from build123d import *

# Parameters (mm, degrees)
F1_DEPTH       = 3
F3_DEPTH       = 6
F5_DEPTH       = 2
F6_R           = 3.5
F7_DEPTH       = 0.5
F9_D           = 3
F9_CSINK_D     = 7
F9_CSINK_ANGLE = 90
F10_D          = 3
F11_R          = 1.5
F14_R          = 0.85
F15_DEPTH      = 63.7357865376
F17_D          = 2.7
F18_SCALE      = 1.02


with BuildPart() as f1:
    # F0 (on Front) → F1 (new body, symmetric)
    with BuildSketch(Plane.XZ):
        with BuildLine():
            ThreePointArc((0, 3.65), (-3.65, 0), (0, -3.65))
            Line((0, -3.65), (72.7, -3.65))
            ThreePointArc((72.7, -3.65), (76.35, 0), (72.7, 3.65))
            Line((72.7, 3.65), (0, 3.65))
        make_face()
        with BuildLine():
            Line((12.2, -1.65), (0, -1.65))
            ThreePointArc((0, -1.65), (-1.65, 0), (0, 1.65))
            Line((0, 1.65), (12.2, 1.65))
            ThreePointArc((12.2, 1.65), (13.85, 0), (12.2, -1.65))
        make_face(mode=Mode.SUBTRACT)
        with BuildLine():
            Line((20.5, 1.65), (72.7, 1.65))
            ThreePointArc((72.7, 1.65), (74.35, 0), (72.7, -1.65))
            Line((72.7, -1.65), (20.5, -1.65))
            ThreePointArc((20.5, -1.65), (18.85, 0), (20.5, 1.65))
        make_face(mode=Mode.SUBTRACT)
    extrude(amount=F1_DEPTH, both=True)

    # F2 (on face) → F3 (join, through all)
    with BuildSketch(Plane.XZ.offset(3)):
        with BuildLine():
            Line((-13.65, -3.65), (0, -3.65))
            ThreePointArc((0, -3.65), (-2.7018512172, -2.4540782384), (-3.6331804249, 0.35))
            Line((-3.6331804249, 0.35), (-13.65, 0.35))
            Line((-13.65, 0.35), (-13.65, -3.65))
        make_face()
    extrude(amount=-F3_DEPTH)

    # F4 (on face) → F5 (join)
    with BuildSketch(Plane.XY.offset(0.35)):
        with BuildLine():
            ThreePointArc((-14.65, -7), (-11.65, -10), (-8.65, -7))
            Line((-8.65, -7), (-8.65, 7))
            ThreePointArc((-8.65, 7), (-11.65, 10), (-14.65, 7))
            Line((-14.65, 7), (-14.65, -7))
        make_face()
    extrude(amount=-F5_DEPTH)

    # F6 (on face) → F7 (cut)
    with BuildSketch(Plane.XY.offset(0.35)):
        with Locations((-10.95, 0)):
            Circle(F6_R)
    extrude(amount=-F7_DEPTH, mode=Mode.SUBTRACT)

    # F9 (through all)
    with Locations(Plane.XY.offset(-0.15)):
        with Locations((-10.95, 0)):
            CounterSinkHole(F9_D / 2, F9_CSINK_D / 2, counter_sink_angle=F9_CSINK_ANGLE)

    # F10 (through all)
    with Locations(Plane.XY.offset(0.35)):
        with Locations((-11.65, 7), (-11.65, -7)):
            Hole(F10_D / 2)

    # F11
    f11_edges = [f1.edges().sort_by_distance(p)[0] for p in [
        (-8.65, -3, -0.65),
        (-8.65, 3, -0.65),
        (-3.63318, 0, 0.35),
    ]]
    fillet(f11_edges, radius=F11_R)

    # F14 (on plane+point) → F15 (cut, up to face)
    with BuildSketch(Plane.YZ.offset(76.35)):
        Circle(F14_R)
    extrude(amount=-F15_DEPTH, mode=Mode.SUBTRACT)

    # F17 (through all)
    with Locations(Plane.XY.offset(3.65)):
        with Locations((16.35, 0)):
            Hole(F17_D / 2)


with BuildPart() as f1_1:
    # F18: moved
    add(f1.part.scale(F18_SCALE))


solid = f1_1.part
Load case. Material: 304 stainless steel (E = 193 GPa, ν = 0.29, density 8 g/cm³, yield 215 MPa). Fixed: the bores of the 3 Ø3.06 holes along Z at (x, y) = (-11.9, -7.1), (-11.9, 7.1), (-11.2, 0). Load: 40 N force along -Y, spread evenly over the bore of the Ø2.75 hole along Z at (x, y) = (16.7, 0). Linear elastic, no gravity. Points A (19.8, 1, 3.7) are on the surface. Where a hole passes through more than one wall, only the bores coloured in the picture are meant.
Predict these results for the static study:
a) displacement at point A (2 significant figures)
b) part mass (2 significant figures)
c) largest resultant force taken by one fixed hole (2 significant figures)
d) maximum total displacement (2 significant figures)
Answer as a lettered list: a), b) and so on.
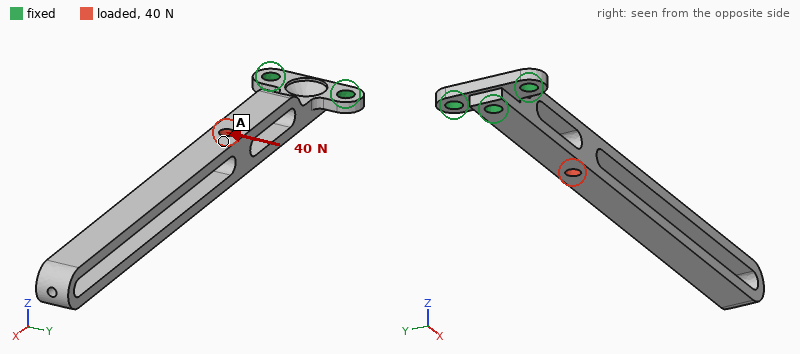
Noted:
a) 26 µm
b) 20 g
c) 81 N
d) 92 µm
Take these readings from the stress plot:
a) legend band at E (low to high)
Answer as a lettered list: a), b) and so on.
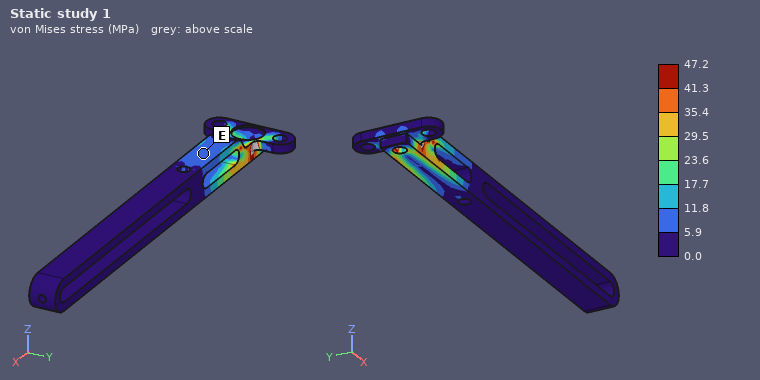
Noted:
a) 5.9 to 11.8 MPa
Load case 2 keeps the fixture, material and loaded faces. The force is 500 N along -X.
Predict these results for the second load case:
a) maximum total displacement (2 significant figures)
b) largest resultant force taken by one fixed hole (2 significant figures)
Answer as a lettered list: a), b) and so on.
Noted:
a) 0.18 mm
b) 210 N
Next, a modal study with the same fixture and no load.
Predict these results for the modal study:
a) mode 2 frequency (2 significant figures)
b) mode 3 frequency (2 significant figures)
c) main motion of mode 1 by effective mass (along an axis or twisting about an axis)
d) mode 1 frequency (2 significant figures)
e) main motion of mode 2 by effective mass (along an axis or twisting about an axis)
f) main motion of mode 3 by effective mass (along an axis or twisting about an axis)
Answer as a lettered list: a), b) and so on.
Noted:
a) 590 Hz
b) 2200 Hz
c) along Z
d) 420 Hz
e) along Y
f) along Z
